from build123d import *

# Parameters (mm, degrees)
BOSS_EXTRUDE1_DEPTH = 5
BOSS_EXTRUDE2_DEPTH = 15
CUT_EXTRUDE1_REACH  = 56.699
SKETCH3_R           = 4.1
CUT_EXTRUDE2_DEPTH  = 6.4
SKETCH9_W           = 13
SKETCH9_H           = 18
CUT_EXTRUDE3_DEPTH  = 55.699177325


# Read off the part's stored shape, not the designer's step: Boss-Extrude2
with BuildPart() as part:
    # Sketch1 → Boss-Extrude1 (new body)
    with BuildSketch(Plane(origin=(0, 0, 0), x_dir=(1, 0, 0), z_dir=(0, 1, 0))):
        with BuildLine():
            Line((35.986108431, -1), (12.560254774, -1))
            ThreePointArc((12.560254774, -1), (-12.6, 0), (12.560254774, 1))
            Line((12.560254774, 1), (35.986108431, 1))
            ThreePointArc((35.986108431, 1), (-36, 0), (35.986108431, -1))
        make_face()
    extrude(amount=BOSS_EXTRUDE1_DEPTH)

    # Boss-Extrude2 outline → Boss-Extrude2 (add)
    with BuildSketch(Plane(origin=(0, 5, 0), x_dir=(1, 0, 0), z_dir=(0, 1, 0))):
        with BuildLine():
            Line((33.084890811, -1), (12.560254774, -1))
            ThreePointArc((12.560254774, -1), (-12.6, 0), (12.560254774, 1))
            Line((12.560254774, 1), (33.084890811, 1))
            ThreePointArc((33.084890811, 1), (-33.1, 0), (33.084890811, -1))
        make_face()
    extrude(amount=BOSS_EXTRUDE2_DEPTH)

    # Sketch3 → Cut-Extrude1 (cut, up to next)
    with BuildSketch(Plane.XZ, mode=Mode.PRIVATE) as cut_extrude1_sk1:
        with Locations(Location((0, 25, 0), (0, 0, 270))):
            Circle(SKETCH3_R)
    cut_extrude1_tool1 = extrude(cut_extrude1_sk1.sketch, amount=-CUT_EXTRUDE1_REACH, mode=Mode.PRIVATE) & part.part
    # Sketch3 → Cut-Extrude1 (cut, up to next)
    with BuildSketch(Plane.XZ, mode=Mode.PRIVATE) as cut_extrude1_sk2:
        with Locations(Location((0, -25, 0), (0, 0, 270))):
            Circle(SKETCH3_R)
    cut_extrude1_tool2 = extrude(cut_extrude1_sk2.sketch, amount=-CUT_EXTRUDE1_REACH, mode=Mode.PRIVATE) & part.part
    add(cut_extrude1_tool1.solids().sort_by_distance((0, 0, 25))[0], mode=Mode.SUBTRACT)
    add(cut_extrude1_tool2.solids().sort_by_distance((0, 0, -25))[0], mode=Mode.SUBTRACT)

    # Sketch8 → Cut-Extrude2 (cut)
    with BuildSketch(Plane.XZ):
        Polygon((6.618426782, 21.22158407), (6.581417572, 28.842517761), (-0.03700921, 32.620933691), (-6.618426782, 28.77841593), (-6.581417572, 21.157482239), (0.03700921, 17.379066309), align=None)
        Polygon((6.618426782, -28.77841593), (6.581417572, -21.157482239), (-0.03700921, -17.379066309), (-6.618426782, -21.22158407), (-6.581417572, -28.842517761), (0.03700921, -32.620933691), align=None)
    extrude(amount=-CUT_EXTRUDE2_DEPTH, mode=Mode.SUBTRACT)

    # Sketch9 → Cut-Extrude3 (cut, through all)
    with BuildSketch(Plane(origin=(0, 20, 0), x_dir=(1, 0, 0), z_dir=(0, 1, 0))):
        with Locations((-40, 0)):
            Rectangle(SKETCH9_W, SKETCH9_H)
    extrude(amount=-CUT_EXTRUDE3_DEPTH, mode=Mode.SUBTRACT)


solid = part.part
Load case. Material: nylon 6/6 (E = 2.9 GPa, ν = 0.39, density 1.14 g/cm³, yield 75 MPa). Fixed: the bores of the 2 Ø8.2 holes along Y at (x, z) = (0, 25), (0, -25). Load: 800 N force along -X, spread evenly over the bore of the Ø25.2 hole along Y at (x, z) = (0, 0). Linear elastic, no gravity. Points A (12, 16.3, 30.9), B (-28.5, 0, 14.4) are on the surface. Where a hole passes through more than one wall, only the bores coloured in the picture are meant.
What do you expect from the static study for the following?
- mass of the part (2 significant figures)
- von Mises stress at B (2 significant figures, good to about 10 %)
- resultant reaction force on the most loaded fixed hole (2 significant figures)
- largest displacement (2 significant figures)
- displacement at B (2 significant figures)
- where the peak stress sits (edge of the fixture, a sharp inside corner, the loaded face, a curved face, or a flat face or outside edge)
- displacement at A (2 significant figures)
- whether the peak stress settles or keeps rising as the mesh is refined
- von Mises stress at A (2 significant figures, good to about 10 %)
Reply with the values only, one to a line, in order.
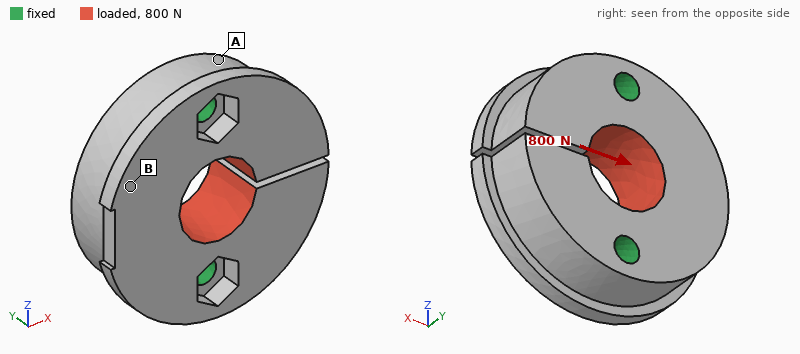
66 g
0.55 MPa
440 N
68 µm
20 µm
edge of the fixture
14 µm
keeps rising
1.2 MPa
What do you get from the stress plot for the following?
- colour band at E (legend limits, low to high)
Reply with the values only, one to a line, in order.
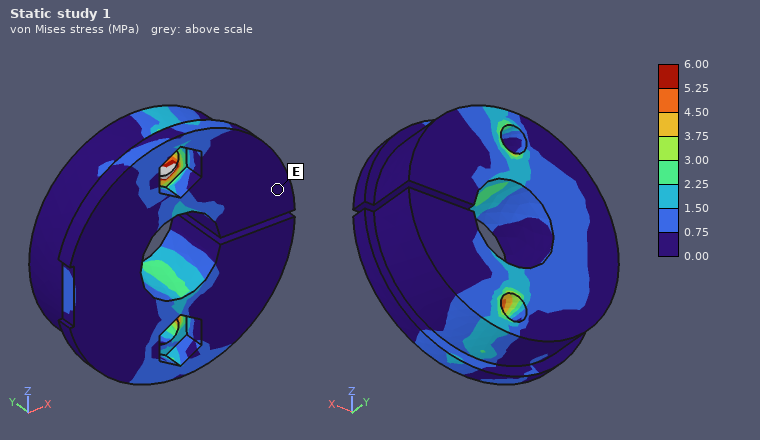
0.00 to 0.75 MPa
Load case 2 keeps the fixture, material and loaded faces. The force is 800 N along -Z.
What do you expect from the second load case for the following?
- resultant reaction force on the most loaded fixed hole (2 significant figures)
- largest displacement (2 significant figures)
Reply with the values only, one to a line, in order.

400 N
18 µm
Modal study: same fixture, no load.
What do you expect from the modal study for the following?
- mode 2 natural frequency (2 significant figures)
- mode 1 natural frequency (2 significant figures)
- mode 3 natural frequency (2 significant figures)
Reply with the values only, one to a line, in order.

2600 Hz
2400 Hz
2800 Hz
